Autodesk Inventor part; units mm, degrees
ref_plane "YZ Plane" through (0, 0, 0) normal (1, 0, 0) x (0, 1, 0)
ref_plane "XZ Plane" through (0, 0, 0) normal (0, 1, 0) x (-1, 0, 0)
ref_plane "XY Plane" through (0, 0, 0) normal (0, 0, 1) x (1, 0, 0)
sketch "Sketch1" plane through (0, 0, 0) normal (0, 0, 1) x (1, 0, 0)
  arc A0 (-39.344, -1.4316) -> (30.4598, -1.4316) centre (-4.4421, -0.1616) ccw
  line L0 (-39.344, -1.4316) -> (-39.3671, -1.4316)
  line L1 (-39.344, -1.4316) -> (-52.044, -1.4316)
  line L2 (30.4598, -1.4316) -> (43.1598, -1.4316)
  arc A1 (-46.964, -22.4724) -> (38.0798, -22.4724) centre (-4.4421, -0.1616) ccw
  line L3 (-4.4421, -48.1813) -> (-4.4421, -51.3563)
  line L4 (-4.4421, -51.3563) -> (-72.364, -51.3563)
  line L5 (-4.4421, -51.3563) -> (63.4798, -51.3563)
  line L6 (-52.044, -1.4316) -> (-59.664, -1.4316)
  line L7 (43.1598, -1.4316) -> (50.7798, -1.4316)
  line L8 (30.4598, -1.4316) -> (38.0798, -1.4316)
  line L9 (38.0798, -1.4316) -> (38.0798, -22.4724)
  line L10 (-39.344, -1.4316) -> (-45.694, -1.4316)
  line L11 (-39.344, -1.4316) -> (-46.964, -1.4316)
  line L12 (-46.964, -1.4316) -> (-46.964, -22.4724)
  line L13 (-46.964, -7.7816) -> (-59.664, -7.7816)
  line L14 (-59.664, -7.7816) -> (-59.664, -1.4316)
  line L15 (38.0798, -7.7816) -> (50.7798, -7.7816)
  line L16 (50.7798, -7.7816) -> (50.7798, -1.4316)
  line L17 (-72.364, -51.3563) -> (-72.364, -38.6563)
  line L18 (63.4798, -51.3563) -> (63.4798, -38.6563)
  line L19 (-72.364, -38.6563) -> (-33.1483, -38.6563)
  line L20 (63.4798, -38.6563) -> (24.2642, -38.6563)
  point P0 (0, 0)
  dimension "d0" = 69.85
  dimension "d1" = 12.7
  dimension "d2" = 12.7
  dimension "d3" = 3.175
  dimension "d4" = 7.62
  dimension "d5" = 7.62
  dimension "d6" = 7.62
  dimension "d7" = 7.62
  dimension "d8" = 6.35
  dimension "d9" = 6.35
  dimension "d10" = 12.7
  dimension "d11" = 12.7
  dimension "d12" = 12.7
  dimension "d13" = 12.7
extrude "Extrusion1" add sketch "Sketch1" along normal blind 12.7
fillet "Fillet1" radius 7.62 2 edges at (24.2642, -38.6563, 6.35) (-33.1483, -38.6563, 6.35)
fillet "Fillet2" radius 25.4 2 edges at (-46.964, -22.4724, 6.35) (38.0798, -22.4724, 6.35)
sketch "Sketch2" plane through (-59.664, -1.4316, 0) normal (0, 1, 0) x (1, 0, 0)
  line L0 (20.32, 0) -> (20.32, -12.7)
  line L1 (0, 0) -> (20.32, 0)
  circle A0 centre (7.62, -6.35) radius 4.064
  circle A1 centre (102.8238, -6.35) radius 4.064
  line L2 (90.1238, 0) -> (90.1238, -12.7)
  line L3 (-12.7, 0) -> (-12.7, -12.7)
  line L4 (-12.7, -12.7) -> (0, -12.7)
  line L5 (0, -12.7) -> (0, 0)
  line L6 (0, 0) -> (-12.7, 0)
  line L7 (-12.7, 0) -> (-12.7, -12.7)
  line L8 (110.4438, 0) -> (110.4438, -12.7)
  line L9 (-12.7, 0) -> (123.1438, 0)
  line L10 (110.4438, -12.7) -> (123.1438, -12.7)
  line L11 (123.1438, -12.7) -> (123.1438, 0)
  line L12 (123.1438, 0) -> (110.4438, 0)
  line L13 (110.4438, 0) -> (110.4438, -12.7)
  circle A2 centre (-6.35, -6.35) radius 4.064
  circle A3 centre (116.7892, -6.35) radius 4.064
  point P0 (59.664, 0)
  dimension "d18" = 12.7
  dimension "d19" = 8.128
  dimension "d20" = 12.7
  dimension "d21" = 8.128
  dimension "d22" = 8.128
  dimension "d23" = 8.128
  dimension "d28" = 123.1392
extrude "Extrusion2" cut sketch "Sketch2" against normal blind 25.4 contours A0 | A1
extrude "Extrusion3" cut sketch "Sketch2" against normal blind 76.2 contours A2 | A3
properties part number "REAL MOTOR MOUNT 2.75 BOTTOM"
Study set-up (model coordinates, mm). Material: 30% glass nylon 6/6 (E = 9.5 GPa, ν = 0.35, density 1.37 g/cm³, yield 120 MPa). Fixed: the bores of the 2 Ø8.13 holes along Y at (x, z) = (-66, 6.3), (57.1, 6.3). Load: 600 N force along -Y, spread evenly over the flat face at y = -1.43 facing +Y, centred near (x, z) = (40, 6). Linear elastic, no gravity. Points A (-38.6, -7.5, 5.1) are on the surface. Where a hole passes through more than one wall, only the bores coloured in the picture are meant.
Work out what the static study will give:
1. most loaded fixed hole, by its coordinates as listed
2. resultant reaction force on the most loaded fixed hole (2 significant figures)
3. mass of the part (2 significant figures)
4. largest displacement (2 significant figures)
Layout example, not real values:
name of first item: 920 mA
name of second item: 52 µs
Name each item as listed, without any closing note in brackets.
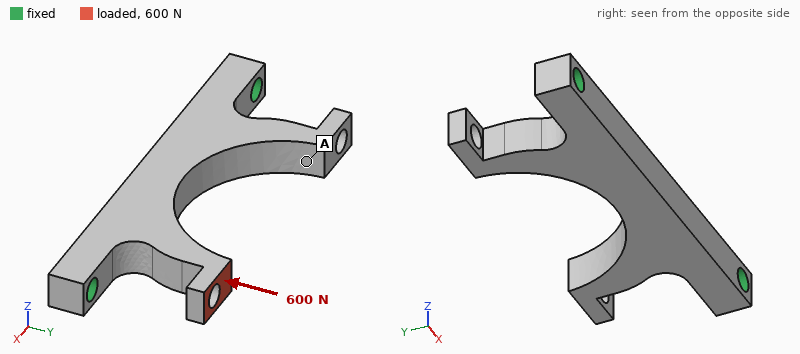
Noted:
most loaded fixed hole, by its coordinates as listed: (57.1, 6.3)
resultant reaction force on the most loaded fixed hole: 580 N
mass of the part: 52 g
largest displacement: 0.47 mm
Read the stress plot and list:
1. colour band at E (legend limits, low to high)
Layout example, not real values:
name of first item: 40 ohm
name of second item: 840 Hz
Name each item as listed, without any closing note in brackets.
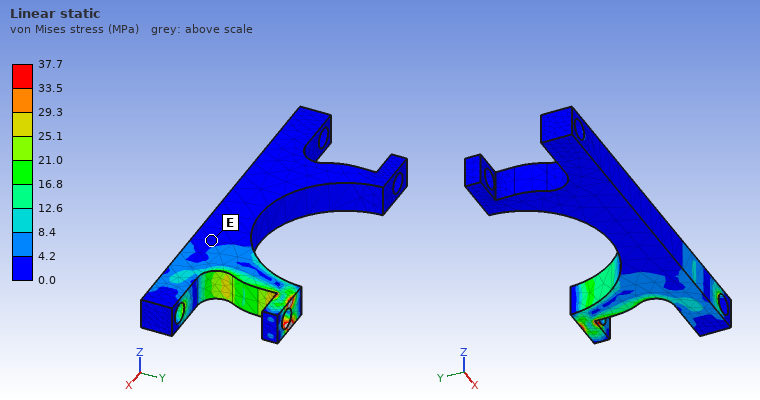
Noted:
colour band at E: 0.0 to 4.2 MPa
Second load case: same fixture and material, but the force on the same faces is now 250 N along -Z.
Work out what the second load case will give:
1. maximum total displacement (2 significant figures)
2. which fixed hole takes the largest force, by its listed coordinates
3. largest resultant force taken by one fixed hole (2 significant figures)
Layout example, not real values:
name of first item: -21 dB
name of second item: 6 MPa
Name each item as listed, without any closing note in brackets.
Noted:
maximum total displacement: 0.92 mm
which fixed hole takes the largest force, by its listed coordinates: (57.1, 6.3)
largest resultant force taken by one fixed hole: 240 N
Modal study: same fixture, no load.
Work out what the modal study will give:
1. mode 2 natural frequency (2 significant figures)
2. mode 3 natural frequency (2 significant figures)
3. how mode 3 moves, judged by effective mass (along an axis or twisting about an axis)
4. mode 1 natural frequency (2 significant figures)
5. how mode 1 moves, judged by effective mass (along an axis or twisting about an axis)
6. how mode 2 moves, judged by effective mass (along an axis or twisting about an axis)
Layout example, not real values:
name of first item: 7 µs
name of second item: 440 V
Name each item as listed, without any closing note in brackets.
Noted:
mode 2 natural frequency: 1900 Hz
mode 3 natural frequency: 2000 Hz
how mode 3 moves, judged by effective mass: along Y
mode 1 natural frequency: 1300 Hz
how mode 1 moves, judged by effective mass: along Z
how mode 2 moves, judged by effective mass: twisting about Y
